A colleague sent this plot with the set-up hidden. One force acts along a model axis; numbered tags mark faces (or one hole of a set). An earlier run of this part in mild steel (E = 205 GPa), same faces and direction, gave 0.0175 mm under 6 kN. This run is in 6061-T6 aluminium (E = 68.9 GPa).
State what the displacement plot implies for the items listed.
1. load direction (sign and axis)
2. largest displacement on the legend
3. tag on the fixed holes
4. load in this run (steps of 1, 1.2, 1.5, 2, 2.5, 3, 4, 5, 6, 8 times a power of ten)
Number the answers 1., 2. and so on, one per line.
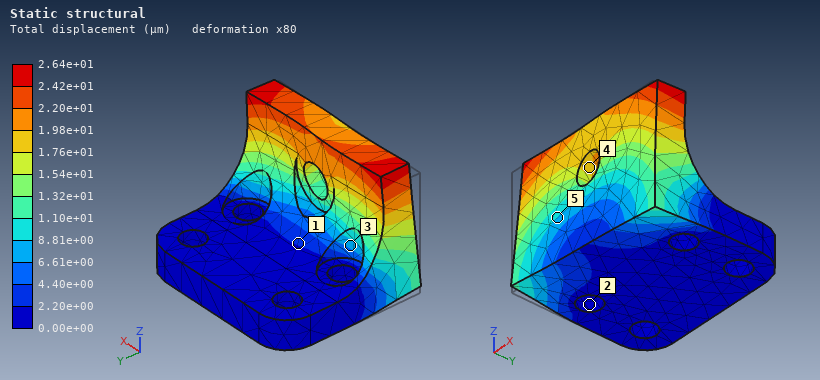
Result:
1. +X
2. 2.64e+01 µm
3. 2
4. 3 kN
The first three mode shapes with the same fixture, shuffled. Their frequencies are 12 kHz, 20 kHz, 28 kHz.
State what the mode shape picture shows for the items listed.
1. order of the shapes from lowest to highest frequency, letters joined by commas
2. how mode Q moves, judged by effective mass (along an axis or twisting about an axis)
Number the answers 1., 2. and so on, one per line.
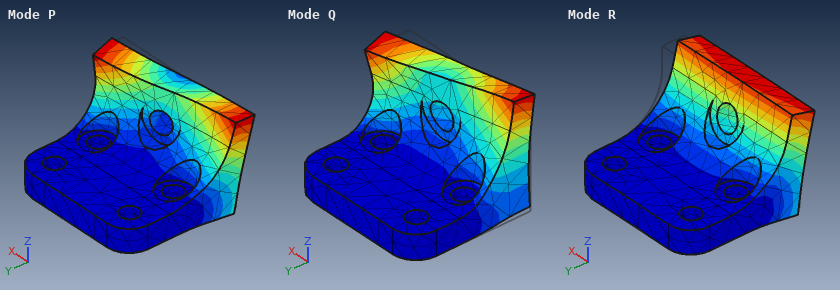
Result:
1. R, P, Q
2. along X
